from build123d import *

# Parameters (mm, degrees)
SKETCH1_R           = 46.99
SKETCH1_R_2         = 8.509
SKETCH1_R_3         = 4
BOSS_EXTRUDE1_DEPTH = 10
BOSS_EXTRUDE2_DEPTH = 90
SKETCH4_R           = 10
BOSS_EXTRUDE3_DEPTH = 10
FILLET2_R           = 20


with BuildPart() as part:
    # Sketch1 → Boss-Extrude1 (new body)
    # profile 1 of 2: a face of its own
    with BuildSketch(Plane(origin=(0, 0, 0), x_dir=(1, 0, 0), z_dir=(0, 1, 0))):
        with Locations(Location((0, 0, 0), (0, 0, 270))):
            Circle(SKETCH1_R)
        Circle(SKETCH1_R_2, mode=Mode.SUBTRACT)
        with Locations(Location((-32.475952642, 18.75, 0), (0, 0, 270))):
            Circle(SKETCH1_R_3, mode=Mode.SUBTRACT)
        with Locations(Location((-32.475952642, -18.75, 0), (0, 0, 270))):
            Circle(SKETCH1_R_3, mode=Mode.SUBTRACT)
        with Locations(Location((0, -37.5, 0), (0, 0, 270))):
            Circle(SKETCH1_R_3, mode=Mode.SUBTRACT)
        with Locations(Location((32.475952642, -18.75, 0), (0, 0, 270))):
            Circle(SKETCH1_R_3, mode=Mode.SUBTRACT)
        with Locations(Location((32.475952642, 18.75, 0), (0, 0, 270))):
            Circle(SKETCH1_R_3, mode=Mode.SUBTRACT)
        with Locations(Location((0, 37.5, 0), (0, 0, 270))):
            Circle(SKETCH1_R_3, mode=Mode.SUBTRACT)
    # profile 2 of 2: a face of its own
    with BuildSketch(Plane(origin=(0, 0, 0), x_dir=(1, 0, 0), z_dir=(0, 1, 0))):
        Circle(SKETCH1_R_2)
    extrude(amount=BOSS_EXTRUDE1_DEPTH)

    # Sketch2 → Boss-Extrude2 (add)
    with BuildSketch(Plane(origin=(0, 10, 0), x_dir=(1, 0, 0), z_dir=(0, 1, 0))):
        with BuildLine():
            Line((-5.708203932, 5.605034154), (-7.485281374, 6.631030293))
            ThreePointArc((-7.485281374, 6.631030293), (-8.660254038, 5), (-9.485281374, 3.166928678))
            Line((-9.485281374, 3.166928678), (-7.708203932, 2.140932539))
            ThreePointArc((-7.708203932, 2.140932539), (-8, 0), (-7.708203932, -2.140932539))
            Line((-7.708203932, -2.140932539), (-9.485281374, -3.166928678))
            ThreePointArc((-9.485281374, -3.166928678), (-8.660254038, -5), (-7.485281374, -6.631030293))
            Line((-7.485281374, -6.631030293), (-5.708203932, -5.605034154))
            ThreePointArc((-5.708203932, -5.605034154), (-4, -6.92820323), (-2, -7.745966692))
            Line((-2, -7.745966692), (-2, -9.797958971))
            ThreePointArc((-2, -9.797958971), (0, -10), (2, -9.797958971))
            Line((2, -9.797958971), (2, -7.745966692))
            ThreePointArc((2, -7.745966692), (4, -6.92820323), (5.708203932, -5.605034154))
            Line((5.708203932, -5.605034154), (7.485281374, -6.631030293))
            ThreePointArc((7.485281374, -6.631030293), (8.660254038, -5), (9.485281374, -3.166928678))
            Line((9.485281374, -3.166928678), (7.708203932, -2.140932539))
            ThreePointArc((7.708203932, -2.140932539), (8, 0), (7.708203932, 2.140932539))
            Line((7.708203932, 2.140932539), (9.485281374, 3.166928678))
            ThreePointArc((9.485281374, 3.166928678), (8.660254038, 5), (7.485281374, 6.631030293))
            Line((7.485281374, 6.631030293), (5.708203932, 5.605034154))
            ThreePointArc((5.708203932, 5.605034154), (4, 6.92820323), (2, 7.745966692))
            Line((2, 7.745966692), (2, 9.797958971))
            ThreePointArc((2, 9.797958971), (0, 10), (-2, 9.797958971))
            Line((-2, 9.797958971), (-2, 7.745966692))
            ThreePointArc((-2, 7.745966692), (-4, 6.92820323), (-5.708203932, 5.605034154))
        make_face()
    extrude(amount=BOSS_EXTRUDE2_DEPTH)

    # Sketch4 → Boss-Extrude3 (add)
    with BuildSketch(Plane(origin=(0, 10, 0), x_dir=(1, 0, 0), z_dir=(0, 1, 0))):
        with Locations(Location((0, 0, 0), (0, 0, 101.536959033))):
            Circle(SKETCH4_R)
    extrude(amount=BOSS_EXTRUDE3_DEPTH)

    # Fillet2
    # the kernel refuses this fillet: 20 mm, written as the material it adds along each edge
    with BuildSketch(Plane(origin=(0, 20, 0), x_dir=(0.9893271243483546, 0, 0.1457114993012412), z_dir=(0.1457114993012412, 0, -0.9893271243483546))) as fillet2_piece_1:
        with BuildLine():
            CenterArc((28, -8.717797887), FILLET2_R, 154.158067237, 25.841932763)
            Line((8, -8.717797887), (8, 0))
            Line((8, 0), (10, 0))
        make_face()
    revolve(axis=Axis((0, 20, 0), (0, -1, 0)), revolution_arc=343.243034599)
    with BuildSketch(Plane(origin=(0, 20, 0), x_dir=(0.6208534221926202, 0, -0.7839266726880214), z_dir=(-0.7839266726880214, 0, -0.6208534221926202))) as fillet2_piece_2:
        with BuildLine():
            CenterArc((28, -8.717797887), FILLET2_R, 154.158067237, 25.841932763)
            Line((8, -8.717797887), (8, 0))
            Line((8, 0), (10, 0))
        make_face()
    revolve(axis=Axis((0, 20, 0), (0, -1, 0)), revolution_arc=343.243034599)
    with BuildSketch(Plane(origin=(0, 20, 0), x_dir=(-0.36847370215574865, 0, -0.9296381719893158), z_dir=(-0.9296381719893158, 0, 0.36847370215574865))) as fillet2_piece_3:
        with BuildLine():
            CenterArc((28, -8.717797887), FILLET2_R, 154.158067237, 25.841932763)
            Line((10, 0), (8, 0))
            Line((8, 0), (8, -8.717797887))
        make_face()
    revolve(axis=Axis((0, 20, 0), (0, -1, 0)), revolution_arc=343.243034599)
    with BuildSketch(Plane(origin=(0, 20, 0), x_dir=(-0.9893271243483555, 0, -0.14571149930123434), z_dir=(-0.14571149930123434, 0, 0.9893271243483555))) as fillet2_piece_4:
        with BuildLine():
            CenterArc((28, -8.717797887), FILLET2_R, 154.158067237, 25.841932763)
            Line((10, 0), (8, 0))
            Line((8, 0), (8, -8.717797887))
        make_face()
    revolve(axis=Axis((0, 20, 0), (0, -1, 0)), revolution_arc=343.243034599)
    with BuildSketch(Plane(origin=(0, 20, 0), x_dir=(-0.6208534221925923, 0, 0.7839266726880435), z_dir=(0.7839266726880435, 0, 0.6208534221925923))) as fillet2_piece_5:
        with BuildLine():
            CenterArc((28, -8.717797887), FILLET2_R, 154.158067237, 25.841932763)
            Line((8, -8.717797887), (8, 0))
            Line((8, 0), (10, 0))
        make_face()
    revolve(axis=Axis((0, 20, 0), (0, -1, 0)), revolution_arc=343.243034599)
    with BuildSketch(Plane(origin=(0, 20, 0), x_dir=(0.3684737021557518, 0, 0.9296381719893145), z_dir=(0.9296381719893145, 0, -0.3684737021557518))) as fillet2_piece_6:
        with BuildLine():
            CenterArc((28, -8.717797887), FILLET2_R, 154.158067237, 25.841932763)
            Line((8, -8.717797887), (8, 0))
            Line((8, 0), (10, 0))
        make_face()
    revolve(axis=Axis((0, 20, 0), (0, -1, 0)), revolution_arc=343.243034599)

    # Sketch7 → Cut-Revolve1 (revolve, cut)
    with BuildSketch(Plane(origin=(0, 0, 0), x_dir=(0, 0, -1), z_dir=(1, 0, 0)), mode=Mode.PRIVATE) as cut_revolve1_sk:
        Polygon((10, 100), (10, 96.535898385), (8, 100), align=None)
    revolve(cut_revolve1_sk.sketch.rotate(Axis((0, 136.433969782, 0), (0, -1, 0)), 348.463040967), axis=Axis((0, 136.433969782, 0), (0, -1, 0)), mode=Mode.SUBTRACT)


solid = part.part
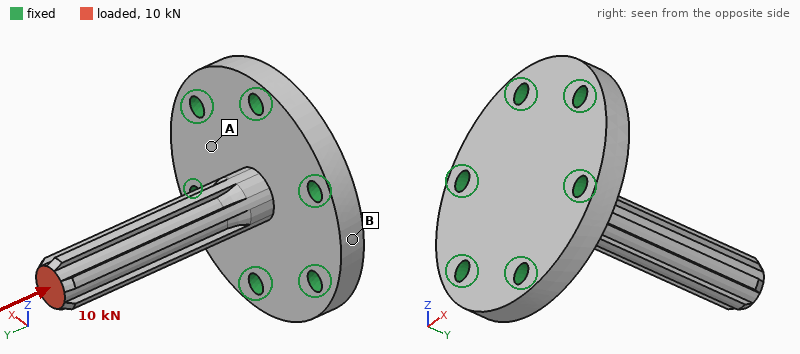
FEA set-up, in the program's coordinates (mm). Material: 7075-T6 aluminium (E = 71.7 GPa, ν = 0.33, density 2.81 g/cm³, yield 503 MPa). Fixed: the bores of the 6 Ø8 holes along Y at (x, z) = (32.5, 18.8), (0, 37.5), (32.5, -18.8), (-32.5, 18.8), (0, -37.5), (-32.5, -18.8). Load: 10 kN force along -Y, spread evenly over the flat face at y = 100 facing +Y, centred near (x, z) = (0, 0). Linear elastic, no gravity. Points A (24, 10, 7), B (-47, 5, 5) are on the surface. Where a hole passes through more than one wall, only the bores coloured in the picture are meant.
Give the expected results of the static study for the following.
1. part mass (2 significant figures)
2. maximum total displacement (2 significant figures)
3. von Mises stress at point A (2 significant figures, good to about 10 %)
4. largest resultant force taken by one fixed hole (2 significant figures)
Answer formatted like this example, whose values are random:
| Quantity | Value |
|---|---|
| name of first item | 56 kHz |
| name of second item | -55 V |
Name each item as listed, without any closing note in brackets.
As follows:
| Quantity | Value |
|---|---|
| part mass | 250 g |
| maximum total displacement | 86 µm |
| von Mises stress at point A | 18 MPa |
| largest resultant force taken by one fixed hole | 1.7 kN |
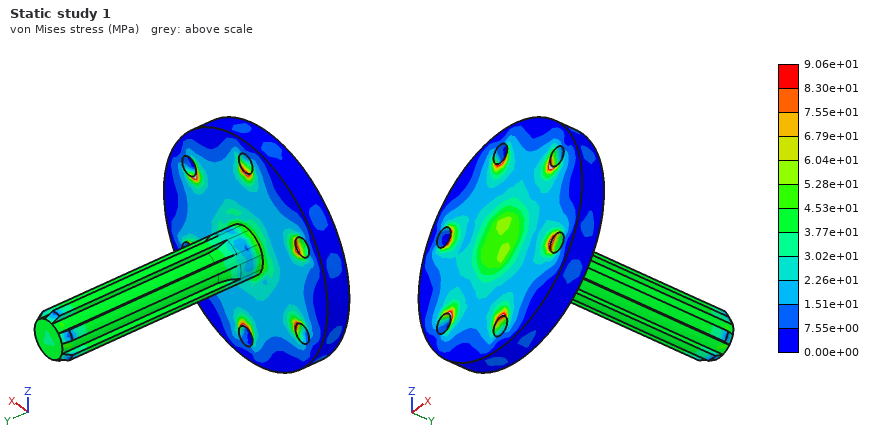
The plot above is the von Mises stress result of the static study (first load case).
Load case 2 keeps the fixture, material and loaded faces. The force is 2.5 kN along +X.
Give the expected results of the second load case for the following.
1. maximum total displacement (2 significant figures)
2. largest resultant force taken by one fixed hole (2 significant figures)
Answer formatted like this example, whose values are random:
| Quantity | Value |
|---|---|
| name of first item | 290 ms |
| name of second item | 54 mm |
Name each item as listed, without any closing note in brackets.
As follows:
| Quantity | Value |
|---|---|
| maximum total displacement | 1.8 mm |
| largest resultant force taken by one fixed hole | 2.5 kN |
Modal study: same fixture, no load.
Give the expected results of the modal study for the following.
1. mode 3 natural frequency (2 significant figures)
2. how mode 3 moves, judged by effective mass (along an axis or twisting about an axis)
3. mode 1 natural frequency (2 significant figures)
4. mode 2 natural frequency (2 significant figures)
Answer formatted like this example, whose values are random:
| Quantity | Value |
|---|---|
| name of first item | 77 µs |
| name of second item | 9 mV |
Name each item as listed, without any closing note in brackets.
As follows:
| Quantity | Value |
|---|---|
| mode 3 natural frequency | 7800 Hz |
| how mode 3 moves, judged by effective mass | along Y |
| mode 1 natural frequency | 1500 Hz |
| mode 2 natural frequency | 1500 Hz |
